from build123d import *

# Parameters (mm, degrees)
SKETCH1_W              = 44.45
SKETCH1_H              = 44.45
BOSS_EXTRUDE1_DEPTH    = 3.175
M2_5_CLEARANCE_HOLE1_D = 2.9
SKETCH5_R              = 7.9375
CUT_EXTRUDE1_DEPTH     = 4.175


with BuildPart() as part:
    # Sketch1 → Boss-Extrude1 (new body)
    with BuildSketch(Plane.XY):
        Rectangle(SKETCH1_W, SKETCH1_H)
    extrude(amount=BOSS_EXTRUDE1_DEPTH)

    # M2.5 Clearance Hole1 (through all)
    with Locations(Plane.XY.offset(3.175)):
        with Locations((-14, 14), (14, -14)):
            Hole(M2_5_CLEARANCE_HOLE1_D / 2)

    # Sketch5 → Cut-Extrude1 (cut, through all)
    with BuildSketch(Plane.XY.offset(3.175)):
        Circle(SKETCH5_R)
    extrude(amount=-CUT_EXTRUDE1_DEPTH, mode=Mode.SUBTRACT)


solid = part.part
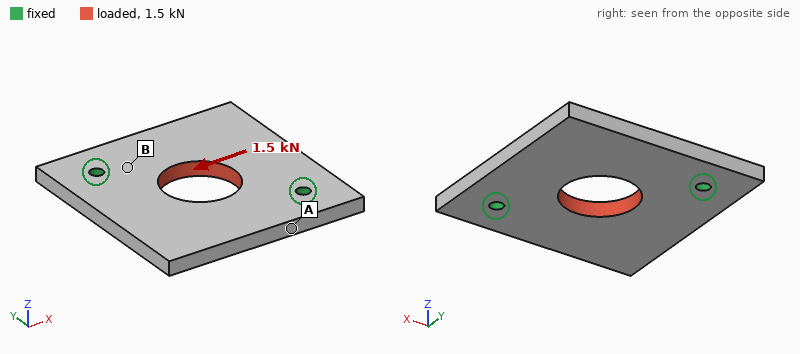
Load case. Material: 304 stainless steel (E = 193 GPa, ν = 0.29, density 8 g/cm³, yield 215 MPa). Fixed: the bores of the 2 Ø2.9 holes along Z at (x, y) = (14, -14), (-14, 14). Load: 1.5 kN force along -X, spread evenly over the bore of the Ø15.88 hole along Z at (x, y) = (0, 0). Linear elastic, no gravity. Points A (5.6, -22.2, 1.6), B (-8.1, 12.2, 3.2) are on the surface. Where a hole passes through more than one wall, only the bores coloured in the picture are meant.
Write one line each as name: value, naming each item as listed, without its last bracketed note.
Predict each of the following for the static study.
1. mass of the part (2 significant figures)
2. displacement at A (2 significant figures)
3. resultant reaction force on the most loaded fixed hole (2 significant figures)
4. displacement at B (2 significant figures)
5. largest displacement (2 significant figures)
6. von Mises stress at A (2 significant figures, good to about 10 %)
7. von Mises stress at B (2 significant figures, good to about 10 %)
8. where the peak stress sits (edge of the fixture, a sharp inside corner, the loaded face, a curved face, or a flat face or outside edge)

mass of the part: 45 g
displacement at A: 0.52 µm
resultant reaction force on the most loaded fixed hole: 750 N
displacement at B: 0.73 µm
largest displacement: 2.0 µm
von Mises stress at A: 7.5 MPa
von Mises stress at B: 19 MPa
where the peak stress sits: edge of the fixture
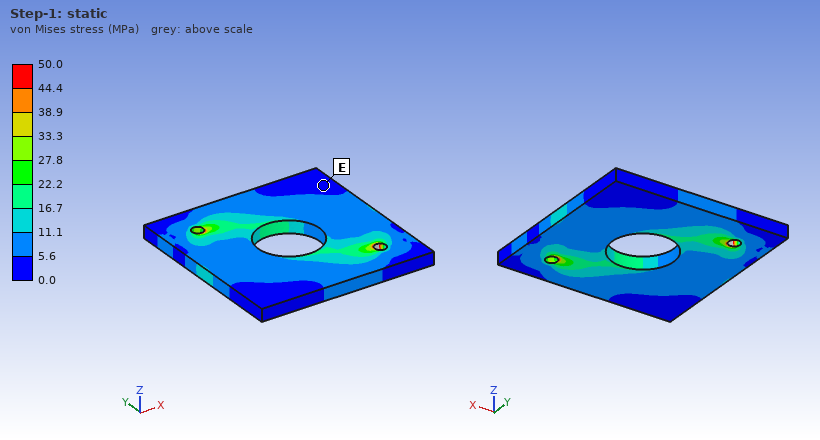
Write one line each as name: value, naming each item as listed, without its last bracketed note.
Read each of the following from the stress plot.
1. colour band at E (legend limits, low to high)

colour band at E: 0.0 to 5.6 MPa
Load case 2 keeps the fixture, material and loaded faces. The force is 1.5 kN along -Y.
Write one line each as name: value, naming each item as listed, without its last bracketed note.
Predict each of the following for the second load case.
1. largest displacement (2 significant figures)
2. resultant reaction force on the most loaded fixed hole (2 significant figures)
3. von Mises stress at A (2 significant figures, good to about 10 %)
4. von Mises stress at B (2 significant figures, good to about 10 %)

largest displacement: 2.0 µm
resultant reaction force on the most loaded fixed hole: 750 N
von Mises stress at A: 7.7 MPa
von Mises stress at B: 12 MPa
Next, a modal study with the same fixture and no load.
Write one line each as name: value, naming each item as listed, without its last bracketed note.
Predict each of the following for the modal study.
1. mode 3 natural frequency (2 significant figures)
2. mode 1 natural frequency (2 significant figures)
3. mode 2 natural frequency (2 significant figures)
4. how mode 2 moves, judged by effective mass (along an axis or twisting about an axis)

mode 3 natural frequency: 11 kHz
mode 1 natural frequency: 3100 Hz
mode 2 natural frequency: 3700 Hz
how mode 2 moves, judged by effective mass: along Z
